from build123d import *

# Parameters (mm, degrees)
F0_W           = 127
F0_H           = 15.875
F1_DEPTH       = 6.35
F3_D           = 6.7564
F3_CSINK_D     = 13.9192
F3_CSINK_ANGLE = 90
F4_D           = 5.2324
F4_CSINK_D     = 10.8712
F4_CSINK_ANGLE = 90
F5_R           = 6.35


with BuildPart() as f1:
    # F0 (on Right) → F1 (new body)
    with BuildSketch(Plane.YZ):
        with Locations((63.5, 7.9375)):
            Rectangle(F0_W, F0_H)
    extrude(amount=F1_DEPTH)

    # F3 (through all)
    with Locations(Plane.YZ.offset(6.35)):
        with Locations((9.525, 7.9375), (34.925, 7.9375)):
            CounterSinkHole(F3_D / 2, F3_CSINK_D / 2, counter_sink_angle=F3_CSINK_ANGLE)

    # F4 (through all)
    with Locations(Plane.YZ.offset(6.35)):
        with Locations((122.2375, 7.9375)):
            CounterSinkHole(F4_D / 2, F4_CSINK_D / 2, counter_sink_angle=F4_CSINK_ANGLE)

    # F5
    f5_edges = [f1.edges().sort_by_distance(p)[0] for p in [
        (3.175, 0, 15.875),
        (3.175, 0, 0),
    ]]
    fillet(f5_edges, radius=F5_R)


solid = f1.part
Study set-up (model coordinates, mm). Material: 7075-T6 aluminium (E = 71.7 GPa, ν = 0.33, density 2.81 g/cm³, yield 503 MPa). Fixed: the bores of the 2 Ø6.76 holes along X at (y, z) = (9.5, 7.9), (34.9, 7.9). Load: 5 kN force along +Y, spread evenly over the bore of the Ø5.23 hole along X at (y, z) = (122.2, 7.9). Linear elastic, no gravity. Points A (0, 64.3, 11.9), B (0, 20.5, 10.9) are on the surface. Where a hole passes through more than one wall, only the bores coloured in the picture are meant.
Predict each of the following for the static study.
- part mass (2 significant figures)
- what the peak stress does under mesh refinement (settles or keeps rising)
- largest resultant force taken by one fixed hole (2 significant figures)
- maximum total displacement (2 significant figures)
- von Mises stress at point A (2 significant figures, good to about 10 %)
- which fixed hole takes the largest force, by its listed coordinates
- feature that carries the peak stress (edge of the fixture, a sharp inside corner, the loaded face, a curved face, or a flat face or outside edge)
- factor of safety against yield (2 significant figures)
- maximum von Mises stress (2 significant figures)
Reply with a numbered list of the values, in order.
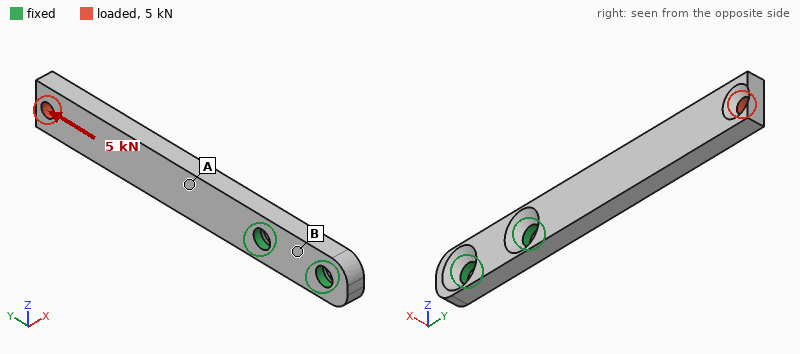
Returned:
1. 33 g
2. settles
3. 4.6 kN
4. 1.1 mm
5. 120 MPa
6. (34.9, 7.9)
7. the loaded face
8. 1.8
9. 280 MPa
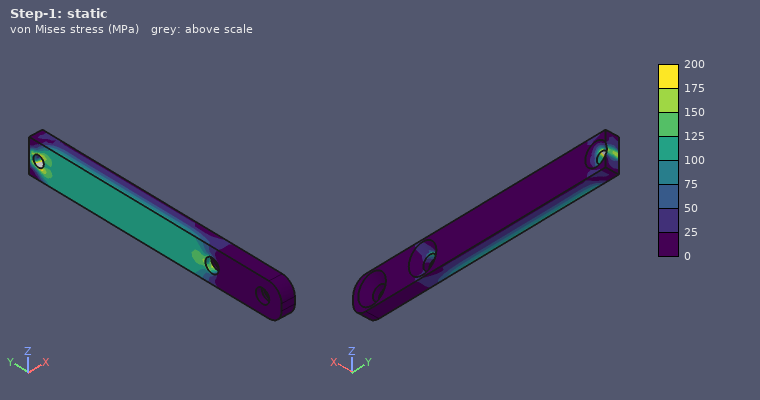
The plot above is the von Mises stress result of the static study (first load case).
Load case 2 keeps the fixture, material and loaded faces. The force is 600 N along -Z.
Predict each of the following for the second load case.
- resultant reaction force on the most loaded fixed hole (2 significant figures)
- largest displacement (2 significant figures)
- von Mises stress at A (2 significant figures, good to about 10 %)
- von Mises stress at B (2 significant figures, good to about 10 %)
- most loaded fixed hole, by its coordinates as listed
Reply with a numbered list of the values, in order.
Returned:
1. 1.5 kN
2. 1.2 mm
3. 68 MPa
4. 31 MPa
5. (34.9, 7.9)
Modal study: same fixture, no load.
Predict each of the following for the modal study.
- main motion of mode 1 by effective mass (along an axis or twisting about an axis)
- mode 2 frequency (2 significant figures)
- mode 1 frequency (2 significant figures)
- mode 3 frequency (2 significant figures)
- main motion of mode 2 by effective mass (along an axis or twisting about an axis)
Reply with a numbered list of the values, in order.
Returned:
1. along X
2. 1400 Hz
3. 580 Hz
4. 3600 Hz
5. along Z
